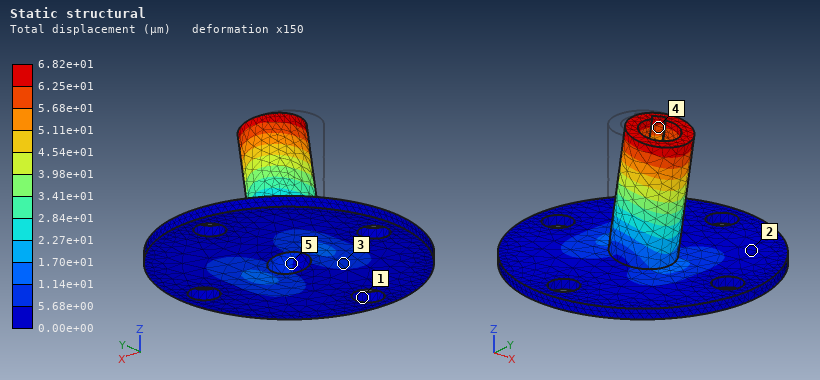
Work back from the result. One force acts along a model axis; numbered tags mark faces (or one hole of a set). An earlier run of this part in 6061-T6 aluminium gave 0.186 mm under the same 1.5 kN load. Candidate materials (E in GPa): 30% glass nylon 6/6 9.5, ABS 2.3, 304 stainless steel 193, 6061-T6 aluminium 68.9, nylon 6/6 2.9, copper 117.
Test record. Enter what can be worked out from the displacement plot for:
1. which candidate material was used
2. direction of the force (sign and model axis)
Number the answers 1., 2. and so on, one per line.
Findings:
1. 304 stainless steel
2. +X
